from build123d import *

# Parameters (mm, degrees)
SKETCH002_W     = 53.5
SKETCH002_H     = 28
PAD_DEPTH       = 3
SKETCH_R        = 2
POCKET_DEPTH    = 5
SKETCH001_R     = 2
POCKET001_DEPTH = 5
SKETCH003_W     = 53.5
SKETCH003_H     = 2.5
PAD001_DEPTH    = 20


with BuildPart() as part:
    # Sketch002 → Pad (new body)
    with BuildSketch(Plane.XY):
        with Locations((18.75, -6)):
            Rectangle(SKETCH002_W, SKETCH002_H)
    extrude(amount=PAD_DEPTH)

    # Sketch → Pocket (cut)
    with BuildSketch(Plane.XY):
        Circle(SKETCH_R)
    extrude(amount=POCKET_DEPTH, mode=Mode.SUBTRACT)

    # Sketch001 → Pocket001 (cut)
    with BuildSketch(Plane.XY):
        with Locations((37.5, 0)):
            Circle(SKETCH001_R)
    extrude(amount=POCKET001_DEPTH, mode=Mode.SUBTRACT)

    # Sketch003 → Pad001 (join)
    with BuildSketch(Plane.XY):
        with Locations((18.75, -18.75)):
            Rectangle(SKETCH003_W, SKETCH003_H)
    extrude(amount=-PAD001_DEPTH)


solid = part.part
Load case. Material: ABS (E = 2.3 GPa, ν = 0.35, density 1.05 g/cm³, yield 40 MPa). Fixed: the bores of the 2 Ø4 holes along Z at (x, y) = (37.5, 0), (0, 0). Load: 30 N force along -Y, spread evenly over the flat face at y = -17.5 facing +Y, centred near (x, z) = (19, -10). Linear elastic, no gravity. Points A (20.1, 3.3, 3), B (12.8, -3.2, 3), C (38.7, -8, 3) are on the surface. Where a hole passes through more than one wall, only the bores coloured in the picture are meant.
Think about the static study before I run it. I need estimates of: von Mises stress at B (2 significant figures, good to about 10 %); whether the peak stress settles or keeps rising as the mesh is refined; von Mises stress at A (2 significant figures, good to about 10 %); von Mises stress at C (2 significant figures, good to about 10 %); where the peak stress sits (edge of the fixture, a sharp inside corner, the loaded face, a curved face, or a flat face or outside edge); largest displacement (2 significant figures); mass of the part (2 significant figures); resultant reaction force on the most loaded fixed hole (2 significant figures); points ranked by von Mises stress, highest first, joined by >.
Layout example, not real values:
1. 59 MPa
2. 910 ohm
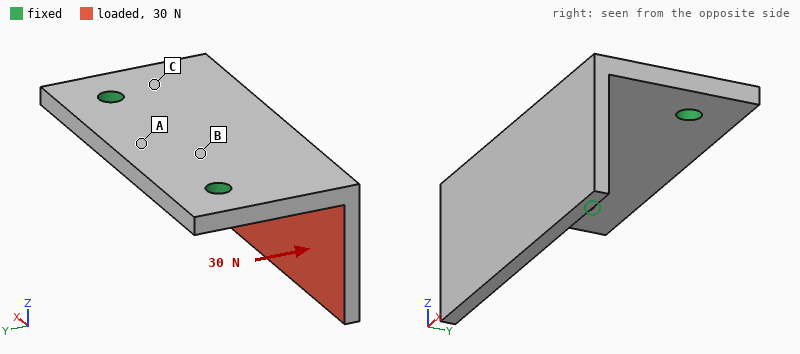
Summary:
1. 2.3 MPa
2. keeps rising
3. 1.1 MPa
4. 4.1 MPa
5. edge of the fixture
6. 0.74 mm
7. 7.4 g
8. 16 N
9. C > B > A
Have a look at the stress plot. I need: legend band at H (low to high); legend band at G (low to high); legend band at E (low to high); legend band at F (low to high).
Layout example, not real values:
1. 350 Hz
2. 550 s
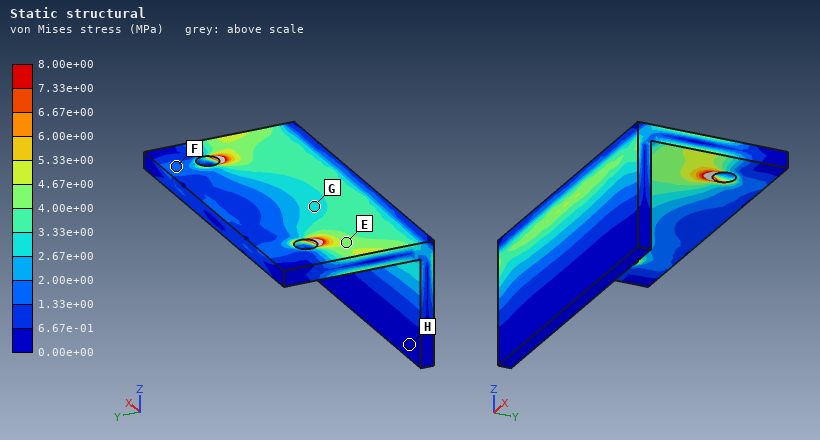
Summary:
1. 0.00e+00 to 6.67e-01 MPa
2. 2.67e+00 to 3.33e+00 MPa
3. 4.00e+00 to 4.67e+00 MPa
4. 1.33e+00 to 2.00e+00 MPa
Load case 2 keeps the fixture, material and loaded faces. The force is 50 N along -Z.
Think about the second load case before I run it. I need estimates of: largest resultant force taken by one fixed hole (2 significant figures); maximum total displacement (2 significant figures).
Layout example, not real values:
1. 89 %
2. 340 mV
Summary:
1. 25 N
2. 0.75 mm
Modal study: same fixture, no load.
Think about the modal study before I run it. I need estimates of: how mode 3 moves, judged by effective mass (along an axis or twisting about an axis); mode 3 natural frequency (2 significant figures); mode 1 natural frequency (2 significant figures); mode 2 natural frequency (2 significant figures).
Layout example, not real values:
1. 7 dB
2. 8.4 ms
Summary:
1. along Z
2. 1500 Hz
3. 610 Hz
4. 1000 Hz
